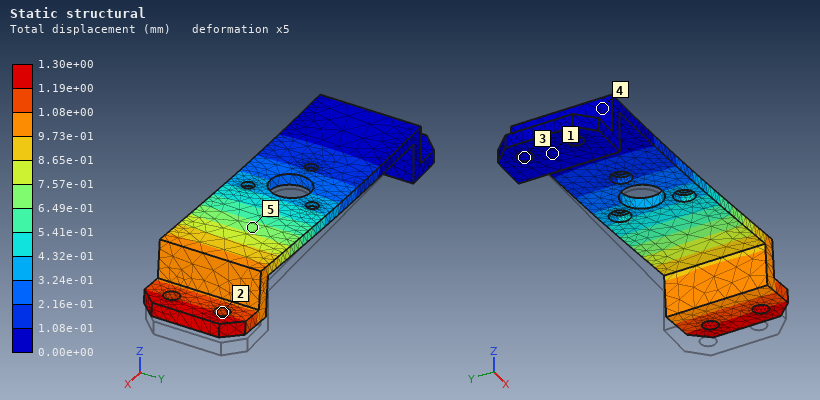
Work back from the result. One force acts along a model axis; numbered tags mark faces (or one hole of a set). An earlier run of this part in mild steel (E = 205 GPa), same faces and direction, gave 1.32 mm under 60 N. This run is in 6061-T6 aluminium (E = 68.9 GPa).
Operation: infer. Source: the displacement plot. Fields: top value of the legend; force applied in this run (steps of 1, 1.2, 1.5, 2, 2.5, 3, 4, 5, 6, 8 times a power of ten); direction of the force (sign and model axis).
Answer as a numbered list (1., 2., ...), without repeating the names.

1. 1.30e+00 mm
2. 20 N
3. +Z
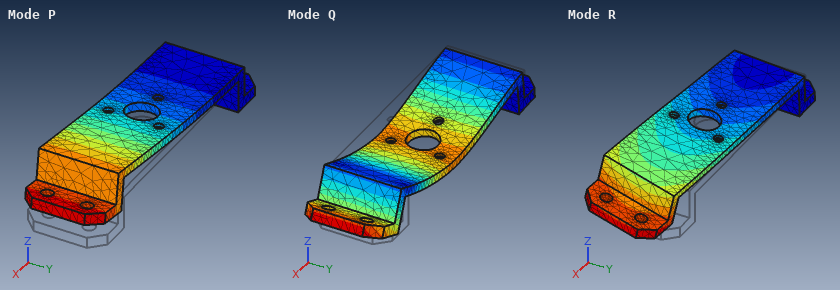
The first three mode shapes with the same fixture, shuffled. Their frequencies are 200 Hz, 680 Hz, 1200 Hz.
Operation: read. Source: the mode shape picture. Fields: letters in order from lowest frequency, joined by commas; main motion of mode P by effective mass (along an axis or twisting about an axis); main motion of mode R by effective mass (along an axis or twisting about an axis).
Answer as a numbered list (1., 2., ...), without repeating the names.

1. P, R, Q
2. along Z
3. along Y
